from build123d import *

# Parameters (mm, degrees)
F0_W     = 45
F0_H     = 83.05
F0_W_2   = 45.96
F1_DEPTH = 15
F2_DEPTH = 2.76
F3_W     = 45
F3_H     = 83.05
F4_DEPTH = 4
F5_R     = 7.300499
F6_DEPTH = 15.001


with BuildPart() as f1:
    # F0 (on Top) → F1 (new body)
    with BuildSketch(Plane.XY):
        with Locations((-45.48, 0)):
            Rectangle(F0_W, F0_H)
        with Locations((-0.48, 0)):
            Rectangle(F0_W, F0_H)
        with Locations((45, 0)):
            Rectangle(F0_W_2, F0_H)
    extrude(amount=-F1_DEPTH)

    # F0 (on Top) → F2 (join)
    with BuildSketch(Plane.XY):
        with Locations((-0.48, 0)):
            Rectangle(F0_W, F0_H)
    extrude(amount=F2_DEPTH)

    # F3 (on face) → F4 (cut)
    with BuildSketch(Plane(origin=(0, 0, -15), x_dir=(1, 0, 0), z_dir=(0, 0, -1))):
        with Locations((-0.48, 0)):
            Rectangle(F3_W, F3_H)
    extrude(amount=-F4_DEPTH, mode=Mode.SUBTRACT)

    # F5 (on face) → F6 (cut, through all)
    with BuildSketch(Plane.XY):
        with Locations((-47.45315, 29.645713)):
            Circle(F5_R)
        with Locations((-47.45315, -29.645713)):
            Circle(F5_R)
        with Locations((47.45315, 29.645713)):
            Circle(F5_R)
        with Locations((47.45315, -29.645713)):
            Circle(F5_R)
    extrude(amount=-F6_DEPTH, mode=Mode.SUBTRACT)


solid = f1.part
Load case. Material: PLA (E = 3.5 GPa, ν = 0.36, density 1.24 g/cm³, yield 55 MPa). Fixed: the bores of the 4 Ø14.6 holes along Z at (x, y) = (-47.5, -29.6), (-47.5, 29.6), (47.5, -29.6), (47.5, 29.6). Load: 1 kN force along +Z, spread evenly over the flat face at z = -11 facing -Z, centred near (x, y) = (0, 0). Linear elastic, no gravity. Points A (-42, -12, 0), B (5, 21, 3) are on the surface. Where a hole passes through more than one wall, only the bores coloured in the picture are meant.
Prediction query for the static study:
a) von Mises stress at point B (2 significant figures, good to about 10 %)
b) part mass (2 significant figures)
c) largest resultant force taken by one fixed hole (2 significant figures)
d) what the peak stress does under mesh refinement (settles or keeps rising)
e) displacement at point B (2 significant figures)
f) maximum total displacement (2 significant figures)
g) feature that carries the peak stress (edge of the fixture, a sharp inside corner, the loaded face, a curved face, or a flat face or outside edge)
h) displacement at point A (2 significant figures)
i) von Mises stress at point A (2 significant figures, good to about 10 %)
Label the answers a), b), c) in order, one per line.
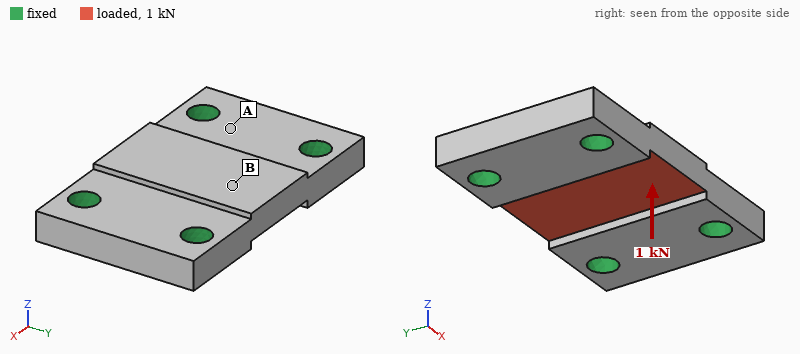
a) 2.0 MPa
b) 190 g
c) 300 N
d) keeps rising
e) 47 µm
f) 51 µm
g) edge of the fixture
h) 8.0 µm
i) 0.94 MPa
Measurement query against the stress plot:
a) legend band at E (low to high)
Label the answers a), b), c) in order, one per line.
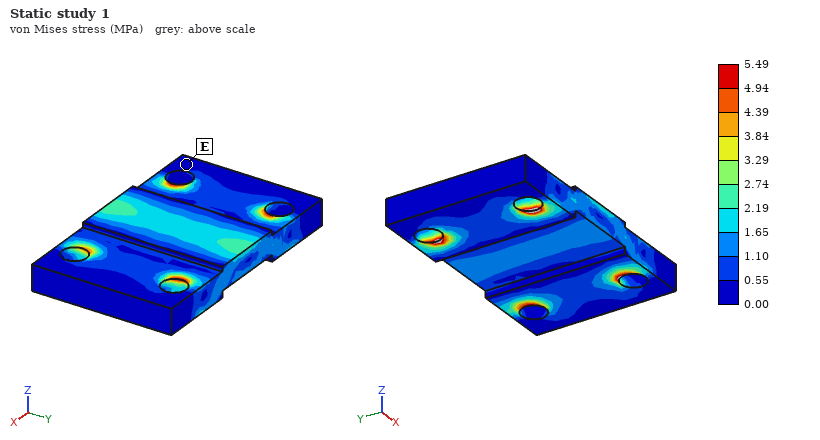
a) 0.00 to 0.55 MPa
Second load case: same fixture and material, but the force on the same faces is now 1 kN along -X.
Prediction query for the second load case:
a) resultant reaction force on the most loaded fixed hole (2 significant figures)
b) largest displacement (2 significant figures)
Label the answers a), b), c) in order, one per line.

a) 260 N
b) 7.7 µm
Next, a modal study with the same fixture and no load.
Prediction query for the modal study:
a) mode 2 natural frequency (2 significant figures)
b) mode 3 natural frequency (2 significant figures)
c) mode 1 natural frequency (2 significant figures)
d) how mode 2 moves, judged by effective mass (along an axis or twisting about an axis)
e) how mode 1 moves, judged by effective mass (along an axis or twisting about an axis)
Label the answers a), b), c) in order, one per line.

a) 3500 Hz
b) 5200 Hz
c) 2800 Hz
d) twisting about X
e) along Z
